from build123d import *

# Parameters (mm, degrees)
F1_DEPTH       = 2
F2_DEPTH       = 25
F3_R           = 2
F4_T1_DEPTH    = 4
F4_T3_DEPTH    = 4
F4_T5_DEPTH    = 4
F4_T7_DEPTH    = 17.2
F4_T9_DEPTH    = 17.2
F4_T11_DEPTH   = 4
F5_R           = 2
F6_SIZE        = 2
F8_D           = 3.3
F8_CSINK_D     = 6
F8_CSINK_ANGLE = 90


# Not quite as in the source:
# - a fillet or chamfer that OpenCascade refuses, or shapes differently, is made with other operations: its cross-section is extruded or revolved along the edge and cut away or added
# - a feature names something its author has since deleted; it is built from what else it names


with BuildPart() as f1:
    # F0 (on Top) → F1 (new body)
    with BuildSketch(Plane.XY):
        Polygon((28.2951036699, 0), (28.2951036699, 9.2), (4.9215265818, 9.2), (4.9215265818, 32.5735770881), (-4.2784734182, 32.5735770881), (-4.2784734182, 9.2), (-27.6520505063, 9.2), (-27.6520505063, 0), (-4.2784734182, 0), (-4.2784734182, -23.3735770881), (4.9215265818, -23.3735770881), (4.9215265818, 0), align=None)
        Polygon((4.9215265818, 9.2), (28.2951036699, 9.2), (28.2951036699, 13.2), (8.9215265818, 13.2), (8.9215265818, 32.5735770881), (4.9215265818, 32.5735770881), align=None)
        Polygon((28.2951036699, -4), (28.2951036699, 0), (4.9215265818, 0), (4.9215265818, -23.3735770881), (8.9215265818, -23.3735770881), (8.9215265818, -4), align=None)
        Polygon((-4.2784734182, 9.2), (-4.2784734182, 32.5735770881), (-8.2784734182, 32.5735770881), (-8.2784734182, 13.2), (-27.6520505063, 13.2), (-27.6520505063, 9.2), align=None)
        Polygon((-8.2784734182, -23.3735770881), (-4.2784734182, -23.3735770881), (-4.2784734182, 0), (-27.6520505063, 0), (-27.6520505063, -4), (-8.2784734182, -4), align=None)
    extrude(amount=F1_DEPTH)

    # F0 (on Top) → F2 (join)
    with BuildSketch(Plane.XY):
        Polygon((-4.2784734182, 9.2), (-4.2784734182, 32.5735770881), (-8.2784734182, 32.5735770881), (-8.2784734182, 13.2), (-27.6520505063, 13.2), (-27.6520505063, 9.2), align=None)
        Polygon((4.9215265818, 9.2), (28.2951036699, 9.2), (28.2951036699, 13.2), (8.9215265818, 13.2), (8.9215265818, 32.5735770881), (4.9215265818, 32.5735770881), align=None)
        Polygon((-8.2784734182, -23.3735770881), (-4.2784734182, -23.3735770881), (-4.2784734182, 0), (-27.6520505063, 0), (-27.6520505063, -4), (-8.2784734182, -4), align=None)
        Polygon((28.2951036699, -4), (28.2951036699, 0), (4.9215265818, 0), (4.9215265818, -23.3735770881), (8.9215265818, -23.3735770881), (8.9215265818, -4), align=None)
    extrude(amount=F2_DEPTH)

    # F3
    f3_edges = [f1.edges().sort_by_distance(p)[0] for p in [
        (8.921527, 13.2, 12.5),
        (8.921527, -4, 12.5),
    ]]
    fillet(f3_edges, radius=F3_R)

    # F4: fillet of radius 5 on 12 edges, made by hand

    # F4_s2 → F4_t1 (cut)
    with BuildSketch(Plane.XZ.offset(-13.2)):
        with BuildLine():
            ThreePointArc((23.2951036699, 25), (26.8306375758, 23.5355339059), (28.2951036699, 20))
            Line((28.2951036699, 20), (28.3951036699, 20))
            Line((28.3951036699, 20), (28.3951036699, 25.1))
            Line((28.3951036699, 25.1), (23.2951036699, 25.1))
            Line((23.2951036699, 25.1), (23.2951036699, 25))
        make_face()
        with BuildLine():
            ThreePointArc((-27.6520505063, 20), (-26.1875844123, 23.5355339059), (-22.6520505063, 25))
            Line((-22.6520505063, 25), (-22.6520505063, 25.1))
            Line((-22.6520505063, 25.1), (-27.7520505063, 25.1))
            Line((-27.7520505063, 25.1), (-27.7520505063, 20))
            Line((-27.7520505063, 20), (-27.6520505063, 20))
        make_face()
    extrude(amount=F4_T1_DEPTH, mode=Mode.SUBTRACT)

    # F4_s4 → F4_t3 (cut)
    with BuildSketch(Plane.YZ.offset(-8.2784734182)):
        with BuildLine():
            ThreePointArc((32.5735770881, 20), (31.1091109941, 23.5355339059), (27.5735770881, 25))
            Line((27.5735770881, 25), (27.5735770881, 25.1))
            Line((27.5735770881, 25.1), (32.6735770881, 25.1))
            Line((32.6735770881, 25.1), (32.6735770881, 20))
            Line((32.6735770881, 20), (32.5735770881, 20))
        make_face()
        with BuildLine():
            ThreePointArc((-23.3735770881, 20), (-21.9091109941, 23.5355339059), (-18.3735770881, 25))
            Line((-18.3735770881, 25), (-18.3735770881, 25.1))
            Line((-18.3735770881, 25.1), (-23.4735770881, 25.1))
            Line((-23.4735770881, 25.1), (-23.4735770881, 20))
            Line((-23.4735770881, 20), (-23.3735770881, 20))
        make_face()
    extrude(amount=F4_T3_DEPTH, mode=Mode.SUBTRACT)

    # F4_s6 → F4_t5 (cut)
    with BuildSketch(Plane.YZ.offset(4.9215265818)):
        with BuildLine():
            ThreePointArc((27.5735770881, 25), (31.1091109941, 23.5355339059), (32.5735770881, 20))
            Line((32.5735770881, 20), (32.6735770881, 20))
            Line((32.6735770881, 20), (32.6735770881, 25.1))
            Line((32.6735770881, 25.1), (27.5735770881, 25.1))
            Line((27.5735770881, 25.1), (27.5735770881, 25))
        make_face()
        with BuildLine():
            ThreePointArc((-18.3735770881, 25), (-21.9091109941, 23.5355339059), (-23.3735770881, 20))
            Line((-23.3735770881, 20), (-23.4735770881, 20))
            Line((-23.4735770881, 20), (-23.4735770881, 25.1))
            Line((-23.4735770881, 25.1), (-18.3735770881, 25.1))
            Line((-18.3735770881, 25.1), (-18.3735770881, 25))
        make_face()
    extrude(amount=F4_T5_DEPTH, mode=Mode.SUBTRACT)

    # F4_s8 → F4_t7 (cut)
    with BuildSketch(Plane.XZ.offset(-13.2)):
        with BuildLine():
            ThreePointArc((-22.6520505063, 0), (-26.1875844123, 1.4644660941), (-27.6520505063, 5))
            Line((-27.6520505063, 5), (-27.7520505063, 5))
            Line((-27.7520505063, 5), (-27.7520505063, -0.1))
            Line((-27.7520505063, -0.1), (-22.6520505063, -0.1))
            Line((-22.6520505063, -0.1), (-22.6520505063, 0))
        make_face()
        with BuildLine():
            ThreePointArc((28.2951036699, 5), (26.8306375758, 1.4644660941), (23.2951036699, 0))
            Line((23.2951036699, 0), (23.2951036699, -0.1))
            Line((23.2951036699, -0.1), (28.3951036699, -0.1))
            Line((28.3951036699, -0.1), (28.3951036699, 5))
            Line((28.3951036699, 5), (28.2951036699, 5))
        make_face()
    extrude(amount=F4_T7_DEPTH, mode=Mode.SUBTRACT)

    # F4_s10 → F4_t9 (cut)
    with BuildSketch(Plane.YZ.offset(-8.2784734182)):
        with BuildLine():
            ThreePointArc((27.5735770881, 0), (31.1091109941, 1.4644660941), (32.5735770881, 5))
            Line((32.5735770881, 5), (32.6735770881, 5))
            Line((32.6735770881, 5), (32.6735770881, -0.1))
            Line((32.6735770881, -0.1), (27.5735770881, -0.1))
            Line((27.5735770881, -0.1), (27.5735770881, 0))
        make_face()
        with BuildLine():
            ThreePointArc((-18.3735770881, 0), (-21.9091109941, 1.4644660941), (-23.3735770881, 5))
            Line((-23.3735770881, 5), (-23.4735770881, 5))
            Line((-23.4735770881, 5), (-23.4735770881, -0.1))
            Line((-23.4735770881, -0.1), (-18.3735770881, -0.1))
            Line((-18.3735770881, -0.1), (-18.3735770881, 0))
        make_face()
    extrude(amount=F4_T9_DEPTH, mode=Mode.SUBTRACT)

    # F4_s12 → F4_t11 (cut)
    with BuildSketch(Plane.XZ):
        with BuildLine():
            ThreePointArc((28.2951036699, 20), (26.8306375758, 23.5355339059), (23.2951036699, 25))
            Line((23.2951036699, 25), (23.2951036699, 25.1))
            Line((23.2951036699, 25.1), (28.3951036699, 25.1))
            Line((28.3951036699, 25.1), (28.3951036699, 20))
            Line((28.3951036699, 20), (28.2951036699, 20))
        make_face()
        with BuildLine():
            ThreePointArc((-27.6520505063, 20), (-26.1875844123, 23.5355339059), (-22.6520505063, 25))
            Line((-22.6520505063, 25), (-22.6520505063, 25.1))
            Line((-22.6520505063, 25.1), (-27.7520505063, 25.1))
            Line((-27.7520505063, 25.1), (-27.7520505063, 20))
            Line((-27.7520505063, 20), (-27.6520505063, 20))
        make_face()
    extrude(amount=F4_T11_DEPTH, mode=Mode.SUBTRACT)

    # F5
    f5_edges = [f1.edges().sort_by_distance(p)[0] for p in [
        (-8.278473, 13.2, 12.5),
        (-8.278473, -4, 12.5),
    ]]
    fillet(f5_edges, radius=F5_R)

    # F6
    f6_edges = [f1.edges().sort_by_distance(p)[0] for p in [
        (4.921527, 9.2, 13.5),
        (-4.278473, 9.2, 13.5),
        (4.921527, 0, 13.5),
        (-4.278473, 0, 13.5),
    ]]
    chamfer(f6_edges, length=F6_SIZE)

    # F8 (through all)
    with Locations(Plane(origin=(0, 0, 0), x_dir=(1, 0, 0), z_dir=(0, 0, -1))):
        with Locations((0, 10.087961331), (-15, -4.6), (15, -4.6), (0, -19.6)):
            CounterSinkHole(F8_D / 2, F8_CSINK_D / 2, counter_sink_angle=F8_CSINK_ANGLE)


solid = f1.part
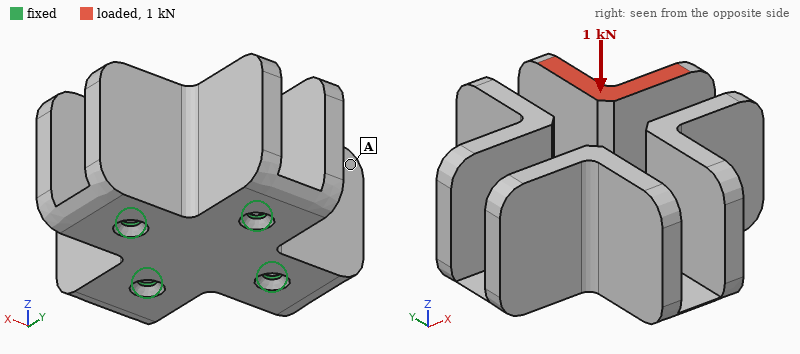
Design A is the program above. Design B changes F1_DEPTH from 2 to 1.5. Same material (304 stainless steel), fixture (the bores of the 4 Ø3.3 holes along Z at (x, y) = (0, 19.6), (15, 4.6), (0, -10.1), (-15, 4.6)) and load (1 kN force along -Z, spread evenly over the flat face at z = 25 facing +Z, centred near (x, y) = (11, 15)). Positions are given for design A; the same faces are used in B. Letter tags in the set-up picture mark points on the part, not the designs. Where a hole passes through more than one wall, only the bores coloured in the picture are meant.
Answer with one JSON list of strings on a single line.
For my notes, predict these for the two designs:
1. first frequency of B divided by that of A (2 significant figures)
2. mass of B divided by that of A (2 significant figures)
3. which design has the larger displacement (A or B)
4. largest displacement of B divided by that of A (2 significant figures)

["0.65", "0.98", "B", "2.2"]
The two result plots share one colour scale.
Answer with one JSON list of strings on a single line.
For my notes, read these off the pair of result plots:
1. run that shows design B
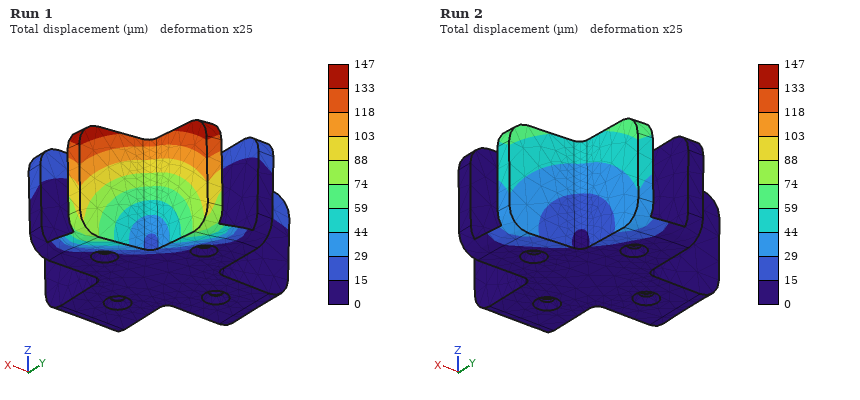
["Run 1"]
